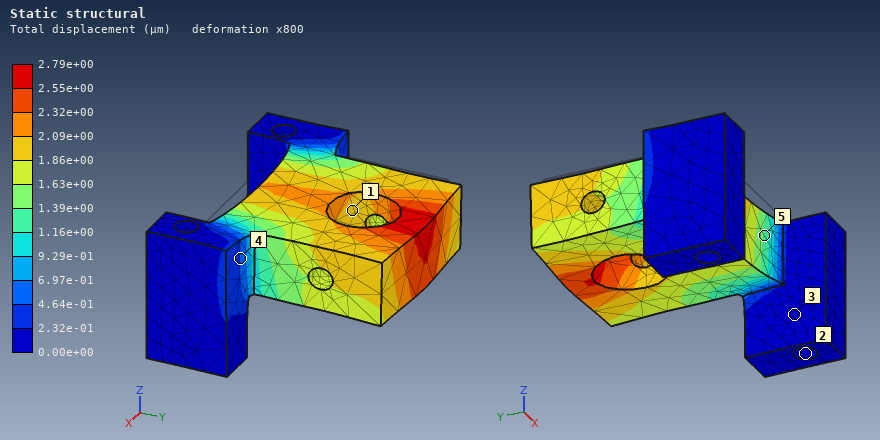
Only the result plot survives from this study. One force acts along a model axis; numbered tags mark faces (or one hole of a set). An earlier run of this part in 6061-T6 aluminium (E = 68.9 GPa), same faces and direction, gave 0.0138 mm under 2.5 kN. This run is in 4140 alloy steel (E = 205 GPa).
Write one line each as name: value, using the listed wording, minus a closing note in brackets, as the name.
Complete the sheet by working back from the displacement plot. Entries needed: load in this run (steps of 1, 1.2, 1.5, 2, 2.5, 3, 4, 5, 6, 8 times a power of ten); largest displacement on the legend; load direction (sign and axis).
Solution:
load in this run: 1.5 kN
largest displacement on the legend: 2.79e+00 µm
load direction: +Y
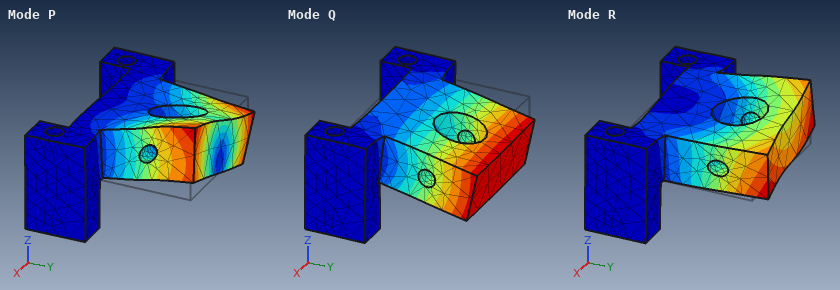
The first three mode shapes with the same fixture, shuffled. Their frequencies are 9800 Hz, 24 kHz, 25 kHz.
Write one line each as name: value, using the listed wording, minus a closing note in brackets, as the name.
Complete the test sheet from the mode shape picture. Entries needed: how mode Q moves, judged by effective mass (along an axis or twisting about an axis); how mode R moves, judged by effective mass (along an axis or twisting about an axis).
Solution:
how mode Q moves, judged by effective mass: along Z
how mode R moves, judged by effective mass: along X
